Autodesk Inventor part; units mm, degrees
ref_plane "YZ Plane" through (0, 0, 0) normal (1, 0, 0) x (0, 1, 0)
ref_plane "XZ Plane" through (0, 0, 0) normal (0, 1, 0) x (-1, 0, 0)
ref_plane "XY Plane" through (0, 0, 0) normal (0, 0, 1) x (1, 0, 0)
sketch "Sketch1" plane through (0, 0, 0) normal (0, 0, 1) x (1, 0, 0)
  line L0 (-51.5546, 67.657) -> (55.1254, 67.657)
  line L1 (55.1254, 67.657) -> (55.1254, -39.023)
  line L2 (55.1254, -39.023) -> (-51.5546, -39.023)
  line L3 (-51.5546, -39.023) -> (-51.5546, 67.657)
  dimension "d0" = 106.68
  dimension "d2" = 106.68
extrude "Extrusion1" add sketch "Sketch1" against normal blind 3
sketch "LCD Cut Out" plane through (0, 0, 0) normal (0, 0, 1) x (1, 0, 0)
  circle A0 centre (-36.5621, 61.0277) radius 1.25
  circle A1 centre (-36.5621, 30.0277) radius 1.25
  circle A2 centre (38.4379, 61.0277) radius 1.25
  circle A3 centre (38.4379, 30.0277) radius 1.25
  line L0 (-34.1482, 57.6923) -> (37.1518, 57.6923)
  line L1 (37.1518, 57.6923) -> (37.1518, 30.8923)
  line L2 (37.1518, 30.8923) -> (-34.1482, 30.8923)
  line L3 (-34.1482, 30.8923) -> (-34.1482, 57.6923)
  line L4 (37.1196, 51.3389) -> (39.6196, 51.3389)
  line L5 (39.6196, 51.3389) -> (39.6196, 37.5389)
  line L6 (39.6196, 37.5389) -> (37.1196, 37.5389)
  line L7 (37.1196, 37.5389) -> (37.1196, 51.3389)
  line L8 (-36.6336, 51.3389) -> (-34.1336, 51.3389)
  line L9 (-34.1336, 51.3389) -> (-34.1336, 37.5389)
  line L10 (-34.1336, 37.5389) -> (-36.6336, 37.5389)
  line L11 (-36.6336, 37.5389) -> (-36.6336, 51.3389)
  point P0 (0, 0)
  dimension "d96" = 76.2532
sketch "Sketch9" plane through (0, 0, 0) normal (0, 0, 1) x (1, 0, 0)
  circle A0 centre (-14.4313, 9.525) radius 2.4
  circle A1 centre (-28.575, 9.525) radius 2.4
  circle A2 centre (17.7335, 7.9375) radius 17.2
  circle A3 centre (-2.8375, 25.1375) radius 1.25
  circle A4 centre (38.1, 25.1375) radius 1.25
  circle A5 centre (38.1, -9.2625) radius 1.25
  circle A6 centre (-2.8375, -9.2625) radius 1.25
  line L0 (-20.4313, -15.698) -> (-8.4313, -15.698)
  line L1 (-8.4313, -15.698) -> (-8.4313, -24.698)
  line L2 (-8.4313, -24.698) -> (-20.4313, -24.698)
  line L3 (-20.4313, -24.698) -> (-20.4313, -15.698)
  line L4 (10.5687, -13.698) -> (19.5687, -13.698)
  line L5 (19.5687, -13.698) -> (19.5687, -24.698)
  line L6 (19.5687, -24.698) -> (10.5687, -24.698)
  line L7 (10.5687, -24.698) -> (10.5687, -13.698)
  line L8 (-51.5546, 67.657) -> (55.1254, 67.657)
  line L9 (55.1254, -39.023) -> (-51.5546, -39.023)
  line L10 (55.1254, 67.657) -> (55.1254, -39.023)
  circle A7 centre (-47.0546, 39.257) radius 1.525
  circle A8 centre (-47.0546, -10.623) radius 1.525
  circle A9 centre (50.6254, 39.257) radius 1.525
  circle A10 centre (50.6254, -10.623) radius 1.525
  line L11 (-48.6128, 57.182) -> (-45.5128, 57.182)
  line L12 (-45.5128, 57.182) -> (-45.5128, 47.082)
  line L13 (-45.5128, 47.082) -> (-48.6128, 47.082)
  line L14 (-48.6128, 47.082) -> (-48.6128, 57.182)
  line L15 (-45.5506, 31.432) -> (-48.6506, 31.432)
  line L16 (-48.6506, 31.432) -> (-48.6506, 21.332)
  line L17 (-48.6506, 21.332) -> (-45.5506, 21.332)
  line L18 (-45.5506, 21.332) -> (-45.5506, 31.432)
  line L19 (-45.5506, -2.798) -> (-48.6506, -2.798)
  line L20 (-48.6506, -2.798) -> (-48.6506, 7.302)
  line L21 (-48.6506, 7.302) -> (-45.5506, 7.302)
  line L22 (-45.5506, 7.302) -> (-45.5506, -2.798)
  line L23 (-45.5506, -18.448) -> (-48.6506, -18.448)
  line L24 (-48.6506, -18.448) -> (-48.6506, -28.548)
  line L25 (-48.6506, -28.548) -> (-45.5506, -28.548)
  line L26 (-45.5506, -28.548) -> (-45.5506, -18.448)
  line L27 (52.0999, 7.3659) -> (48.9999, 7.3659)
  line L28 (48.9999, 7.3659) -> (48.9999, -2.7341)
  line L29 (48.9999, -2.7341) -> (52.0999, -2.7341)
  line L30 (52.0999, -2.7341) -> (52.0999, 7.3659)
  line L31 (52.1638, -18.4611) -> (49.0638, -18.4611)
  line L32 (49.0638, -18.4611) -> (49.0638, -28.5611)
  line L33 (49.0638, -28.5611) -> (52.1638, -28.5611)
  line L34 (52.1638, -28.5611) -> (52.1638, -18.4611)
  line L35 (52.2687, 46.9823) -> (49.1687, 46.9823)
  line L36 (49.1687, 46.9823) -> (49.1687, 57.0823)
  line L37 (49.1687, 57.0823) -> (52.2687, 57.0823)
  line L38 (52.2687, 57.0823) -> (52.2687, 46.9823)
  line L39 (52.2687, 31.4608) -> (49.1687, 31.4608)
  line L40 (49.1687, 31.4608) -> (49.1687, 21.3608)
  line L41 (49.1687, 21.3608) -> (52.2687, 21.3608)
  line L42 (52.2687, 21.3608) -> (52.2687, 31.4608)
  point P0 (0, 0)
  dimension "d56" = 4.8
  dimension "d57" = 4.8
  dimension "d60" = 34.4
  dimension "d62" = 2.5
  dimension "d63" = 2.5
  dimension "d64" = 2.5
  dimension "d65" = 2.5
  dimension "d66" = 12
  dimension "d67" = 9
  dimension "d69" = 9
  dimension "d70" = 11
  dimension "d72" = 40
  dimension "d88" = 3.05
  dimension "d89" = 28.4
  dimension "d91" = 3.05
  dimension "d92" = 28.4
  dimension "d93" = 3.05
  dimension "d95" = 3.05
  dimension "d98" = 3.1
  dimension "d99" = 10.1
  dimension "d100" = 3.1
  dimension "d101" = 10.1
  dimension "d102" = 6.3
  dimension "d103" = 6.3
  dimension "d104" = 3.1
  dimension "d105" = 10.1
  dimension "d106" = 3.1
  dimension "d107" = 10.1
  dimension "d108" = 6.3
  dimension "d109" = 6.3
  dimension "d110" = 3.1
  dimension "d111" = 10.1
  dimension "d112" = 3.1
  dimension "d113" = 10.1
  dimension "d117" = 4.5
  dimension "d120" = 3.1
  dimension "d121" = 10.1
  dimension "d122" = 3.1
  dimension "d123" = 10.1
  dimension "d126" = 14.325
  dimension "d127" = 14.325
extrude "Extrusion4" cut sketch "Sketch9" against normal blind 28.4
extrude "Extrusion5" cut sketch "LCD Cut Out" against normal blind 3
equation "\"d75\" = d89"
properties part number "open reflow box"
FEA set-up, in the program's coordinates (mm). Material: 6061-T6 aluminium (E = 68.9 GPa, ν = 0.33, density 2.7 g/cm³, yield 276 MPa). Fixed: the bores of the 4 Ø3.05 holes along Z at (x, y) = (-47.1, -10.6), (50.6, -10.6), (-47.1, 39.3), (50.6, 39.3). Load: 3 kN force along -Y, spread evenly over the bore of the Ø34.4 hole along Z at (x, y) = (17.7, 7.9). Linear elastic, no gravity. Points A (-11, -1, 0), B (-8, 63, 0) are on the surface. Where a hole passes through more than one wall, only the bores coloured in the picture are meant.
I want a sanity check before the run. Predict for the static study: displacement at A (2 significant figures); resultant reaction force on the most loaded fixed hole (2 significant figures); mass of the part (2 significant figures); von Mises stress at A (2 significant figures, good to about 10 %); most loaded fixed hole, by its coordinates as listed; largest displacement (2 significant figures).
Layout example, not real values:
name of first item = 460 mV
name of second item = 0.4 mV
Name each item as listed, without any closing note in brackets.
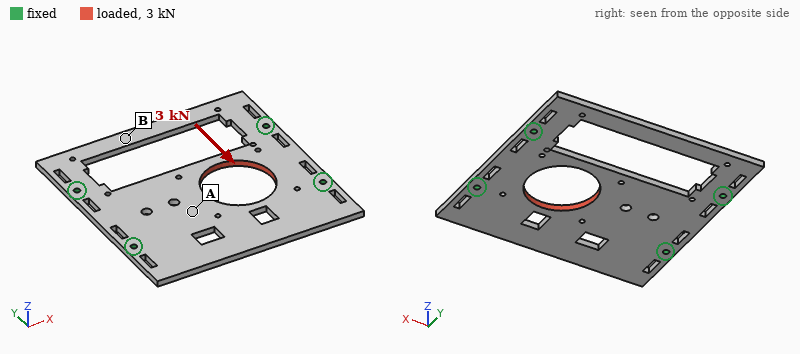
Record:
displacement at A = 19 µm
resultant reaction force on the most loaded fixed hole = 1.2 kN
mass of the part = 64 g
von Mises stress at A = 16 MPa
most loaded fixed hole, by its coordinates as listed = (50.6, -10.6)
largest displacement = 39 µm
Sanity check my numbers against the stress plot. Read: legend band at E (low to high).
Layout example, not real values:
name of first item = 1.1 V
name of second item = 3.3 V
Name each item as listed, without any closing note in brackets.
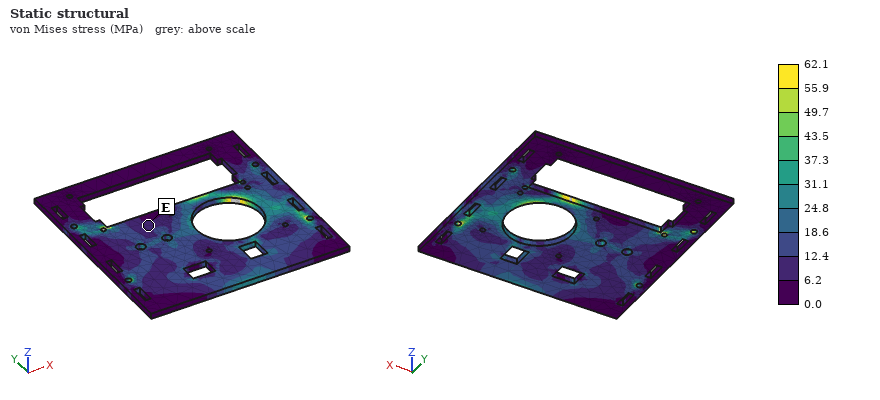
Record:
legend band at E = 6.2 to 12.4 MPa
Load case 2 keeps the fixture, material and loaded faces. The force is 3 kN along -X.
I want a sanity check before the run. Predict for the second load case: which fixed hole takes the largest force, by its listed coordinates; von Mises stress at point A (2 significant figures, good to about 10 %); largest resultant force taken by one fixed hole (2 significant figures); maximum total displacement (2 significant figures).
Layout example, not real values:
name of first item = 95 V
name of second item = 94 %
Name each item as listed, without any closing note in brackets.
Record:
which fixed hole takes the largest force, by its listed coordinates = (50.6, -10.6)
von Mises stress at point A = 9.2 MPa
largest resultant force taken by one fixed hole = 1.3 kN
maximum total displacement = 17 µm
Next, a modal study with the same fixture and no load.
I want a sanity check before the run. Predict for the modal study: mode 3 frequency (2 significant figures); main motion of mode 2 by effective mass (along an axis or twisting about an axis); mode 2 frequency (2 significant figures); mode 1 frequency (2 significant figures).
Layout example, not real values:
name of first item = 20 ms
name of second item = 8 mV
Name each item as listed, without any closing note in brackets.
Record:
mode 3 frequency = 1600 Hz
main motion of mode 2 by effective mass = along Z
mode 2 frequency = 1200 Hz
mode 1 frequency = 1100 Hz
